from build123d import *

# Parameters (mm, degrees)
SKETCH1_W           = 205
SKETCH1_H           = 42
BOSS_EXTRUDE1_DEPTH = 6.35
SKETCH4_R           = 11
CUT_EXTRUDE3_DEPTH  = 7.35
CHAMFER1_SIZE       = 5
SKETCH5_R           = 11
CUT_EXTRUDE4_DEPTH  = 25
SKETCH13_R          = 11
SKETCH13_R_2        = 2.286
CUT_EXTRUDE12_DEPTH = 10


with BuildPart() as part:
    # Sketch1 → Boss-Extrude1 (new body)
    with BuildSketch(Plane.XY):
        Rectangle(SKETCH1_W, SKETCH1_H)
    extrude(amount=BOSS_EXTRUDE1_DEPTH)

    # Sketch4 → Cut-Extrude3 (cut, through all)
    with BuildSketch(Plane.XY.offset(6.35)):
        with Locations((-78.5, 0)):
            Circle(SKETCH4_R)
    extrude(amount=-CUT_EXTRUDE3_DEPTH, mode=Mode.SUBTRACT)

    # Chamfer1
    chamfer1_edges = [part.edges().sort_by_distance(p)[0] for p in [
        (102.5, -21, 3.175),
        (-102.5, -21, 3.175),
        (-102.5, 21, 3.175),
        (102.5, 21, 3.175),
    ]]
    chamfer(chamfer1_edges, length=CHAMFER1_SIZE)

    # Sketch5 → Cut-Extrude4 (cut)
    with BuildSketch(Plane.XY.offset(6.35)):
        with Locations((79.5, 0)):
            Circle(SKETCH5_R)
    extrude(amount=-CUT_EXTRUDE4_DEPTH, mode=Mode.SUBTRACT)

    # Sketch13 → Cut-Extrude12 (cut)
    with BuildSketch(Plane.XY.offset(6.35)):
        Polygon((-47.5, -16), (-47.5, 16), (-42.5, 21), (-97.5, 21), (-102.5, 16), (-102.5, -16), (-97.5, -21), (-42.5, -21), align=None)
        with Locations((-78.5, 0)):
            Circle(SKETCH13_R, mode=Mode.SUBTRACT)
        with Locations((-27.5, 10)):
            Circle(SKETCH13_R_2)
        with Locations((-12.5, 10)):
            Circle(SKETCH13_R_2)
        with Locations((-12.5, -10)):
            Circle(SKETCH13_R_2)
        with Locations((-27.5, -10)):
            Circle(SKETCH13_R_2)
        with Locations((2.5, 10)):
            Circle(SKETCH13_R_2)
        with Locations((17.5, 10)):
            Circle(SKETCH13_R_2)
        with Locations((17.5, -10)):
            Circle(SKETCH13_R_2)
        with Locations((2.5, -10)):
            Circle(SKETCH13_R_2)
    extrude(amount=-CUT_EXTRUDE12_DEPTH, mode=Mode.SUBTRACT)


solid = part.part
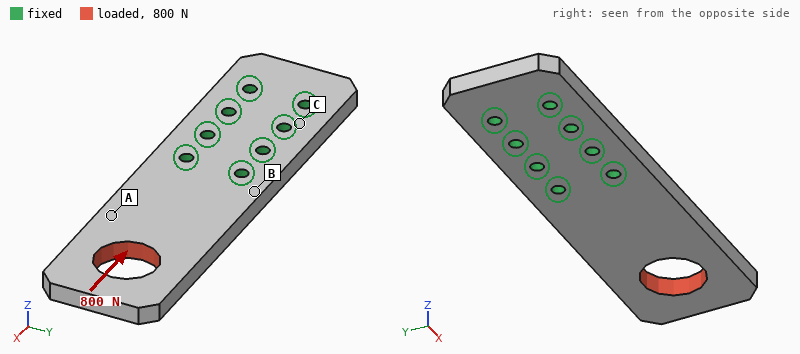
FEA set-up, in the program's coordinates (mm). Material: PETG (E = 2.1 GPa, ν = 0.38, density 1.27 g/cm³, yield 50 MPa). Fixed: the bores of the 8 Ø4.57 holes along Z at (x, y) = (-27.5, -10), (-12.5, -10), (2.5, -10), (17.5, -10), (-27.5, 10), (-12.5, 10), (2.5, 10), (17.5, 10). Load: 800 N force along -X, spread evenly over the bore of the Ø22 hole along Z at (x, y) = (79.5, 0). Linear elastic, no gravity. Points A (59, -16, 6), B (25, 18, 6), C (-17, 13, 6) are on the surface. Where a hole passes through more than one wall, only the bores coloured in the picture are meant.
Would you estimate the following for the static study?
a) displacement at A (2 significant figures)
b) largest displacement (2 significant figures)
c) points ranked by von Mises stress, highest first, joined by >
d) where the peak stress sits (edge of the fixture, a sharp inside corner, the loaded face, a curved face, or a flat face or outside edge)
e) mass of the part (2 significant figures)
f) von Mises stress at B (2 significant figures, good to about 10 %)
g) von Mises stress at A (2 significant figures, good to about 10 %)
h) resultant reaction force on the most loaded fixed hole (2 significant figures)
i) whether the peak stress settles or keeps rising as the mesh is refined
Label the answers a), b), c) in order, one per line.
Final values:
a) 0.067 mm
b) 0.16 mm
c) A > B > C
d) edge of the fixture
e) 46 g
f) 2.3 MPa
g) 3.6 MPa
h) 320 N
i) keeps rising
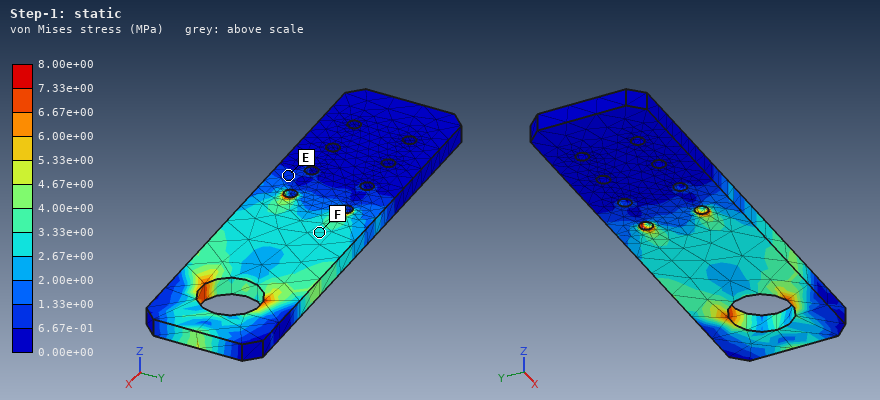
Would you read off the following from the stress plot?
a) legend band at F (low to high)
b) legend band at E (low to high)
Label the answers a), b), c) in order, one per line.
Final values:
a) 2.67e+00 to 3.33e+00 MPa
b) 6.67e-01 to 1.33e+00 MPa
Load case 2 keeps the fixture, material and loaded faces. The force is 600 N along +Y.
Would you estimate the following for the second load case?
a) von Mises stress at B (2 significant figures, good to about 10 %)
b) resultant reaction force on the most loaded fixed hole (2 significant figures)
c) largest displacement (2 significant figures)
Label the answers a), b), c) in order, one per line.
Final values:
a) 13 MPa
b) 1.2 kN
c) 1.5 mm
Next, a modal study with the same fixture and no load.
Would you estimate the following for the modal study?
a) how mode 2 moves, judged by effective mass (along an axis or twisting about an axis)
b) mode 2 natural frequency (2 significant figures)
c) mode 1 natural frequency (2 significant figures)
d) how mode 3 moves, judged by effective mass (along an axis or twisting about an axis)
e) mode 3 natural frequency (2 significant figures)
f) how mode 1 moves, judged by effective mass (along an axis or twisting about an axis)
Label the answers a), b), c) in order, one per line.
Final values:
a) twisting about X
b) 720 Hz
c) 210 Hz
d) along Y
e) 990 Hz
f) along Z
